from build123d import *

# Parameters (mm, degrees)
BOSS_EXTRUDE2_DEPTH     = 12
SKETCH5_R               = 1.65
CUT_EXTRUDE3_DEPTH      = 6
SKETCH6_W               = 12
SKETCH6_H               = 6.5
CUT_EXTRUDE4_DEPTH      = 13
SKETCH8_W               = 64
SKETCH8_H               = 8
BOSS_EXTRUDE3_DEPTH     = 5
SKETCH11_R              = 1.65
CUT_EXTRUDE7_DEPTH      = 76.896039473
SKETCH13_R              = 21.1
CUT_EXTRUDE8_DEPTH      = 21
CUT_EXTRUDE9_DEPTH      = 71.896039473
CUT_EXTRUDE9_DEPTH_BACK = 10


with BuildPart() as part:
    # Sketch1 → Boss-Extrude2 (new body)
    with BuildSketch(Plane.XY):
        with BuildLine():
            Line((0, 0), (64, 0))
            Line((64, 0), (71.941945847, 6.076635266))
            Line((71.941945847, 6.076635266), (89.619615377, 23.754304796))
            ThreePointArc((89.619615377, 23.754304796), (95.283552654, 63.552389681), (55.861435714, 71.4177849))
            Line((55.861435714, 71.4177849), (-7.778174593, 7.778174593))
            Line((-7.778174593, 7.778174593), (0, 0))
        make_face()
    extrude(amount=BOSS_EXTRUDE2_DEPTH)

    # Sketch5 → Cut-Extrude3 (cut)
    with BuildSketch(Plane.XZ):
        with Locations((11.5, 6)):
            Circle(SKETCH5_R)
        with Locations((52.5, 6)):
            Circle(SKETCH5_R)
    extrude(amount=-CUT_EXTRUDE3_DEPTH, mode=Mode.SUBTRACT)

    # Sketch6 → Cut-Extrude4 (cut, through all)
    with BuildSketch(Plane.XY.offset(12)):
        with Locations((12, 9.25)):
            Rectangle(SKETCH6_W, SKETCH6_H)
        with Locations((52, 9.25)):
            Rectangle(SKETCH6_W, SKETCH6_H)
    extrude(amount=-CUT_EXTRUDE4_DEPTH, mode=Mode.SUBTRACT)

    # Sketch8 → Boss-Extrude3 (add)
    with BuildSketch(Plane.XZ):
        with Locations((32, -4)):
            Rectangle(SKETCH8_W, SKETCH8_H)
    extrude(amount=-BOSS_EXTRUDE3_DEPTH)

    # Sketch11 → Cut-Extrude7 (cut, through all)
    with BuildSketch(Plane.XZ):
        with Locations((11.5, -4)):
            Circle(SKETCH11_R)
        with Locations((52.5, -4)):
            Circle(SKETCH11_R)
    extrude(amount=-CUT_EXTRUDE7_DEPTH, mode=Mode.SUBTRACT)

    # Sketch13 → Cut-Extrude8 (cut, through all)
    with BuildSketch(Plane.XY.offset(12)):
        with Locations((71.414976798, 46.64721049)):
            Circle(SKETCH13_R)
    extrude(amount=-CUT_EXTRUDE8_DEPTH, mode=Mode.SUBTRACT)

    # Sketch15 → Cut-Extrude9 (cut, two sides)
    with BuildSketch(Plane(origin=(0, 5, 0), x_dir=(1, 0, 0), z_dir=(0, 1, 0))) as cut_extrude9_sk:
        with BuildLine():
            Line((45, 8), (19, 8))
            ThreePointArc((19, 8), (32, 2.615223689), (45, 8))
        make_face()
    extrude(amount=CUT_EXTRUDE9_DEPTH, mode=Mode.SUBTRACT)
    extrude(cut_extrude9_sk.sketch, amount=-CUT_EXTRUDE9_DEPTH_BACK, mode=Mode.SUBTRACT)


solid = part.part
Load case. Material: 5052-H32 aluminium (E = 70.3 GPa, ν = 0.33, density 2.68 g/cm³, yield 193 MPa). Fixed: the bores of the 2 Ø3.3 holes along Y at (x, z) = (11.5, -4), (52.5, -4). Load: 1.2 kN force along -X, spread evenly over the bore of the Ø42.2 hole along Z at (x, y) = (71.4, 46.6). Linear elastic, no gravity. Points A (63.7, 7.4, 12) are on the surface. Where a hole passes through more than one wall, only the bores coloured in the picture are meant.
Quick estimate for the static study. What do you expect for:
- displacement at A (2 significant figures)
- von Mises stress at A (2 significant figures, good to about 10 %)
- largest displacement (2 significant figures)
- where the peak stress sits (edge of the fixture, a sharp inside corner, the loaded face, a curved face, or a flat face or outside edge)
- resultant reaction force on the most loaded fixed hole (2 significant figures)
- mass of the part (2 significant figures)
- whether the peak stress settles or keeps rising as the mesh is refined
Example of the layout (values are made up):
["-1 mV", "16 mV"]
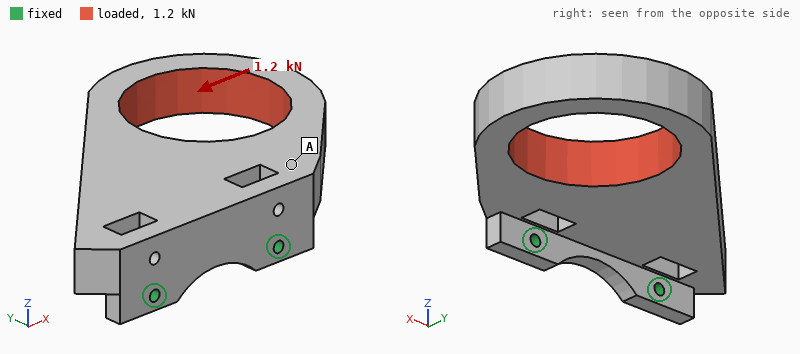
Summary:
["0.029 mm", "9.7 MPa", "0.11 mm", "edge of the fixture", "1.4 kN", "120 g", "keeps rising"]
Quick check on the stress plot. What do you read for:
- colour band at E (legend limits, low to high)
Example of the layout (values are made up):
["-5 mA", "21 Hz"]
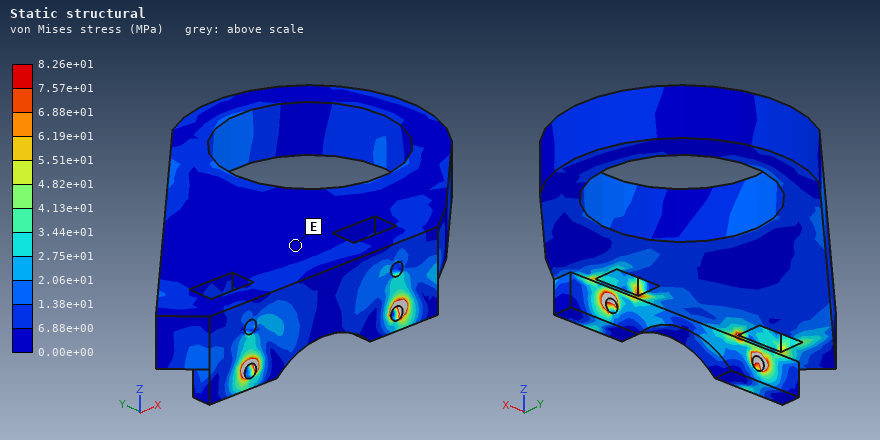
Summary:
["0.00e+00 to 6.88e+00 MPa"]
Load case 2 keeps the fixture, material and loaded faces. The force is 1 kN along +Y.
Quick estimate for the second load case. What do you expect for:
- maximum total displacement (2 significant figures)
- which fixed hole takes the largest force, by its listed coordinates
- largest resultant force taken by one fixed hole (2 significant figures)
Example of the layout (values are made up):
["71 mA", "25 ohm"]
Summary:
["0.19 mm", "(52.5, -4)", "1.4 kN"]
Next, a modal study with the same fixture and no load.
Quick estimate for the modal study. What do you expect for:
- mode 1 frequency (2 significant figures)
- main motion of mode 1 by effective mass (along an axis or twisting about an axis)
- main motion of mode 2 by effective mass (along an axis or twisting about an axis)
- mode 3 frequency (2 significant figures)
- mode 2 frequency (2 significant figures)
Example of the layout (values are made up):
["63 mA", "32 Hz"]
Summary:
["770 Hz", "along Z", "along X", "3000 Hz", "2400 Hz"]
